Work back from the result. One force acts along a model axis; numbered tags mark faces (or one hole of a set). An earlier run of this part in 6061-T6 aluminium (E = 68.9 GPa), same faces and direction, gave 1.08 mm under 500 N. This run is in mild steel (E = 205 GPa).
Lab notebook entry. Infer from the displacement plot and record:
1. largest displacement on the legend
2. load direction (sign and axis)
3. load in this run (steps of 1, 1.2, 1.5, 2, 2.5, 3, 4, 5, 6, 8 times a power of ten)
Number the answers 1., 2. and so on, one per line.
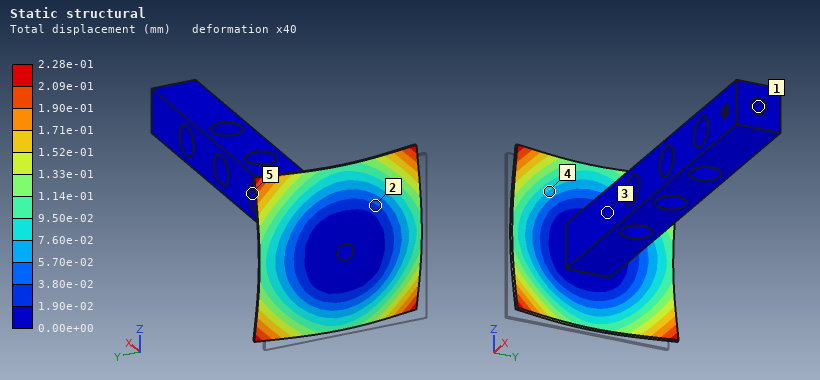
1. 2.28e-01 mm
2. +X
3. 300 N
